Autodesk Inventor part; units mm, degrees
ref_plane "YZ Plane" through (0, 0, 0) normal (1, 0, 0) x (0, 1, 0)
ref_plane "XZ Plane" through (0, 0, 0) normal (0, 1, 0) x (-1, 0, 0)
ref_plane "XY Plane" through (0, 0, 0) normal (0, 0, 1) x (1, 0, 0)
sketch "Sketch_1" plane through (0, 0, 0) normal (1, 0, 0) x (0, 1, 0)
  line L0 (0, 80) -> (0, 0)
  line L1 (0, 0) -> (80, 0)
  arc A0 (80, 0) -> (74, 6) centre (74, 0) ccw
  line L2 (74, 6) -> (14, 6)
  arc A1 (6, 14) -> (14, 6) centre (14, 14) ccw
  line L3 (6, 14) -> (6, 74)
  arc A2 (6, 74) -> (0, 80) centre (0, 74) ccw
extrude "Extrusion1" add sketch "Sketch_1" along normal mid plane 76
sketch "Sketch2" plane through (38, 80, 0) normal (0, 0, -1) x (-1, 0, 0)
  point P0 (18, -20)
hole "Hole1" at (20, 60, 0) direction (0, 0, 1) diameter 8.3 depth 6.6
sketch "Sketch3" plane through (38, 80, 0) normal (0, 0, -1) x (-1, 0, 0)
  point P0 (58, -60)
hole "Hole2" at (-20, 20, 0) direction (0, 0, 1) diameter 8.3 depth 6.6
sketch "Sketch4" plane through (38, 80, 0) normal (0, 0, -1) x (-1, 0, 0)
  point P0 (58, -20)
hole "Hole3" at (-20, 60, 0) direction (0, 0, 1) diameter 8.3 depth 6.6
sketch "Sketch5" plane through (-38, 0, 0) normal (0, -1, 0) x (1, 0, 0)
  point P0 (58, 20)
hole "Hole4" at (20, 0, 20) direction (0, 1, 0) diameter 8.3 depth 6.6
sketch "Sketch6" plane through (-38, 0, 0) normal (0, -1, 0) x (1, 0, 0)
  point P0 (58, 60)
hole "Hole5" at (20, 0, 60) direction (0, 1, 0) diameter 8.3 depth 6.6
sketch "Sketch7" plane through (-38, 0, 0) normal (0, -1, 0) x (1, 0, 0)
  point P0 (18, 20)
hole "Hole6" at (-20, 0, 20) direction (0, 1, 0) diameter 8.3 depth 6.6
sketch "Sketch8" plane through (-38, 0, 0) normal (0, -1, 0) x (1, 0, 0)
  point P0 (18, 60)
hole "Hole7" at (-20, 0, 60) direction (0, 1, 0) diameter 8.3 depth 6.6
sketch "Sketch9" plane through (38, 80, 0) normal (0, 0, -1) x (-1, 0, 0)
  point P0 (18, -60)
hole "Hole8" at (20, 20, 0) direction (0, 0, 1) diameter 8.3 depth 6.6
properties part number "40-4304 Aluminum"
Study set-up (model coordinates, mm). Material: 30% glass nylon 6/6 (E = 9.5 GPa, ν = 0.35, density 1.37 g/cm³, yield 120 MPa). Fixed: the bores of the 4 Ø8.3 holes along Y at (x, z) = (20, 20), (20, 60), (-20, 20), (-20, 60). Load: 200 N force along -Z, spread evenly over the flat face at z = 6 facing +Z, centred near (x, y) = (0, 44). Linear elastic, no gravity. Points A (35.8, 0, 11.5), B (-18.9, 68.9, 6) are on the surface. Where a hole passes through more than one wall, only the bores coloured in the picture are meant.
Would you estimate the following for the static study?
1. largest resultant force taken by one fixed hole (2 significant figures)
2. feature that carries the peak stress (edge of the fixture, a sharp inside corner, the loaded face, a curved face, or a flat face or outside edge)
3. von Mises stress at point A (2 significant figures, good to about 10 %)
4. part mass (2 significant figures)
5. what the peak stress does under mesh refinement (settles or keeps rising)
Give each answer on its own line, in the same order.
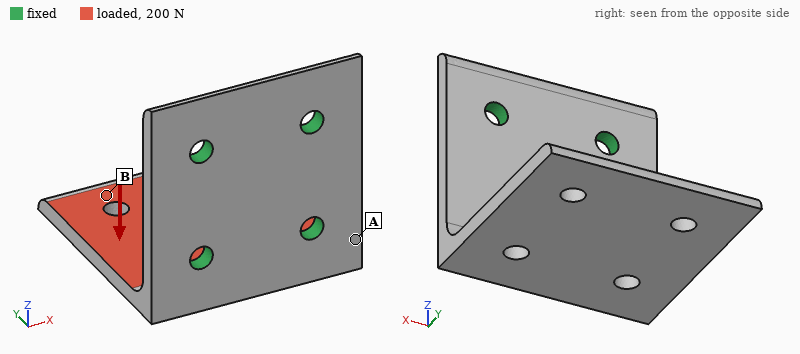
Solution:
93 N
edge of the fixture
11 MPa
92 g
keeps rising
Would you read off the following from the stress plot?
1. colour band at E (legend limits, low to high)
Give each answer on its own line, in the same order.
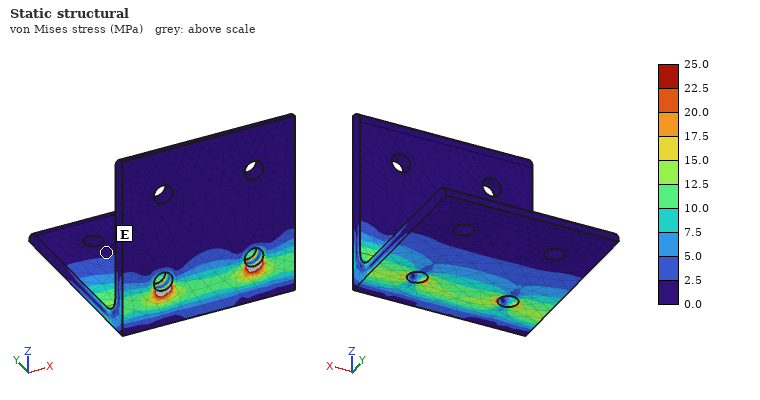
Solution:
0.0 to 2.5 MPa
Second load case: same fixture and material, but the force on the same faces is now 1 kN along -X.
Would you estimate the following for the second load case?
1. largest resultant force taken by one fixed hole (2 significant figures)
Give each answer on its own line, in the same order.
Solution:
1.1 kN
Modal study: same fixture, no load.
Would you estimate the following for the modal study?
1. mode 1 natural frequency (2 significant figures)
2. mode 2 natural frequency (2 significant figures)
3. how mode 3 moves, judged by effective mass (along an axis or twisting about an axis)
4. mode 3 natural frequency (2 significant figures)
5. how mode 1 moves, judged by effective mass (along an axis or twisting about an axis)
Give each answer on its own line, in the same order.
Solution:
390 Hz
950 Hz
along X
1400 Hz
along Z
